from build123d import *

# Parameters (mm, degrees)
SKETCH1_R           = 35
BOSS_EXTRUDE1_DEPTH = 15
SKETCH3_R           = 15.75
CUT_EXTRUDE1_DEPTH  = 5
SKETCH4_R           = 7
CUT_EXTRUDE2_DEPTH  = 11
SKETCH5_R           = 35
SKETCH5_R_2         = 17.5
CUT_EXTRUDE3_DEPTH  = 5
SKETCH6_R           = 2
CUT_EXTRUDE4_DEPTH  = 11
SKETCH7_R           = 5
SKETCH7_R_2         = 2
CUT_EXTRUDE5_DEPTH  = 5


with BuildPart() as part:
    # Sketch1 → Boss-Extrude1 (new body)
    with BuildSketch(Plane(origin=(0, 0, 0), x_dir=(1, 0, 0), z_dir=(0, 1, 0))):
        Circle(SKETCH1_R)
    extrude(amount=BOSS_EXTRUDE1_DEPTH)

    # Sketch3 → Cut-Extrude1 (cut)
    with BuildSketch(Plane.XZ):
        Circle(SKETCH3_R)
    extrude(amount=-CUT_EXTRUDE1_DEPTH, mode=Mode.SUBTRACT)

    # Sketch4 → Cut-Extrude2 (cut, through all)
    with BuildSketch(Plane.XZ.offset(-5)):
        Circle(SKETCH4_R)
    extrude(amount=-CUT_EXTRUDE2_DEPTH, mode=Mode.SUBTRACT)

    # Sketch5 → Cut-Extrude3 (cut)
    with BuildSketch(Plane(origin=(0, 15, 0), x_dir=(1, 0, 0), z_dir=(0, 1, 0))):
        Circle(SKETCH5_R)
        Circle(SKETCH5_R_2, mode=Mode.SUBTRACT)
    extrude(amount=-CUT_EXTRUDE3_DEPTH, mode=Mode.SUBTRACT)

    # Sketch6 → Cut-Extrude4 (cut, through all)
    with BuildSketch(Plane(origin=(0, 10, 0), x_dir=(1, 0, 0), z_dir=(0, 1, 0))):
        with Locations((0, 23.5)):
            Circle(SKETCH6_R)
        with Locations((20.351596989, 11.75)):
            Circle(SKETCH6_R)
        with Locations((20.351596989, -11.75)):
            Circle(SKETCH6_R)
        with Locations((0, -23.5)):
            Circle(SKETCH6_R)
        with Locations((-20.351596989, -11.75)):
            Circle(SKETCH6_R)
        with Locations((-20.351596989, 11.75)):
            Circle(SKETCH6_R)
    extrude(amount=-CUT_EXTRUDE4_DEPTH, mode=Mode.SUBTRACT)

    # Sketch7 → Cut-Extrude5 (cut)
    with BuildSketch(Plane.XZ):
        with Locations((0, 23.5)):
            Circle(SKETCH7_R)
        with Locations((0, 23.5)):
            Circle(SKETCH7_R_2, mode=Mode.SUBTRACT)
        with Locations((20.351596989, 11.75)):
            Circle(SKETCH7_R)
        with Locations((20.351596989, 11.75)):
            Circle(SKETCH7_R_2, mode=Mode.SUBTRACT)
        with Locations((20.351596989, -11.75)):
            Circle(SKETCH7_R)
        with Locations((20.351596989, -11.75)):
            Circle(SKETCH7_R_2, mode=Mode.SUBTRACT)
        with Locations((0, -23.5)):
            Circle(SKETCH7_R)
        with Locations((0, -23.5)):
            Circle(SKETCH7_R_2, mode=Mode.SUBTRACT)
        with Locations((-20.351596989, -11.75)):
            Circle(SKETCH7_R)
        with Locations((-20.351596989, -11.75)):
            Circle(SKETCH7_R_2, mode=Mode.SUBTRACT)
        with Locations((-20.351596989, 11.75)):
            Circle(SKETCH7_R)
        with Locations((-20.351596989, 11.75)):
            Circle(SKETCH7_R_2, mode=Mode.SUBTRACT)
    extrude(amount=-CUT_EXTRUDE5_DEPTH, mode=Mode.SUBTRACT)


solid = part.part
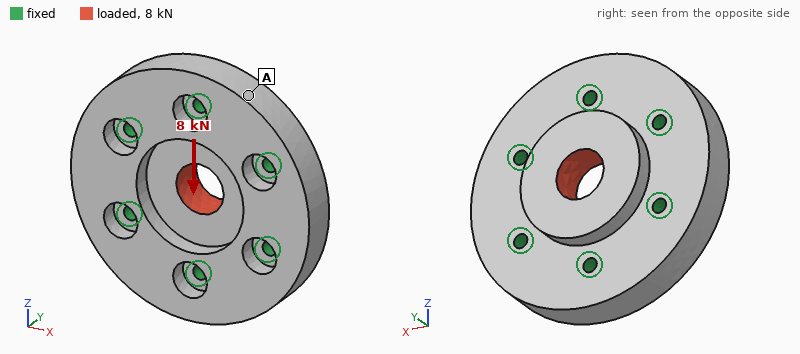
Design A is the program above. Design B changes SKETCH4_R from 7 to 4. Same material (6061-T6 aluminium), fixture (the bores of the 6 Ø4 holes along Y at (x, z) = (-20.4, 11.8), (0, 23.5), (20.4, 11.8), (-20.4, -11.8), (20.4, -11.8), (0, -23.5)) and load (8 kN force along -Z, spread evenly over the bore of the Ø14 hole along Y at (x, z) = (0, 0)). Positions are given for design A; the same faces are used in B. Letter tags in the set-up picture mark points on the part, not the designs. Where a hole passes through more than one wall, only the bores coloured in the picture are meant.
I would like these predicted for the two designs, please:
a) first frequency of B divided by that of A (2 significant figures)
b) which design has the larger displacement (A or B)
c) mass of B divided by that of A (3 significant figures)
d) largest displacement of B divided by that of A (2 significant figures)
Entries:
1.00
B
1.03
1.1
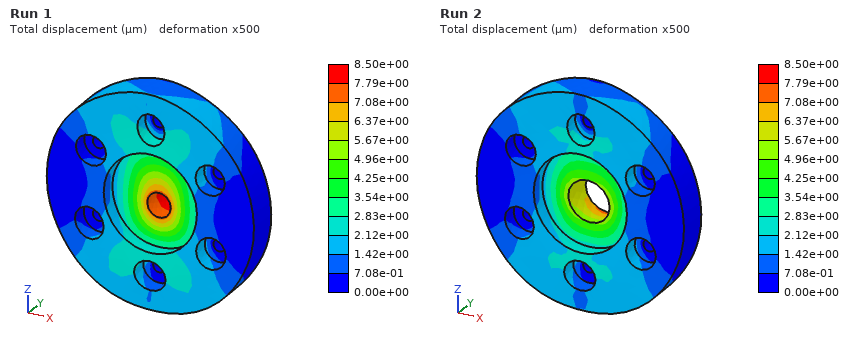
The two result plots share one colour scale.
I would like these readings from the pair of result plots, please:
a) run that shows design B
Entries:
Run 1
